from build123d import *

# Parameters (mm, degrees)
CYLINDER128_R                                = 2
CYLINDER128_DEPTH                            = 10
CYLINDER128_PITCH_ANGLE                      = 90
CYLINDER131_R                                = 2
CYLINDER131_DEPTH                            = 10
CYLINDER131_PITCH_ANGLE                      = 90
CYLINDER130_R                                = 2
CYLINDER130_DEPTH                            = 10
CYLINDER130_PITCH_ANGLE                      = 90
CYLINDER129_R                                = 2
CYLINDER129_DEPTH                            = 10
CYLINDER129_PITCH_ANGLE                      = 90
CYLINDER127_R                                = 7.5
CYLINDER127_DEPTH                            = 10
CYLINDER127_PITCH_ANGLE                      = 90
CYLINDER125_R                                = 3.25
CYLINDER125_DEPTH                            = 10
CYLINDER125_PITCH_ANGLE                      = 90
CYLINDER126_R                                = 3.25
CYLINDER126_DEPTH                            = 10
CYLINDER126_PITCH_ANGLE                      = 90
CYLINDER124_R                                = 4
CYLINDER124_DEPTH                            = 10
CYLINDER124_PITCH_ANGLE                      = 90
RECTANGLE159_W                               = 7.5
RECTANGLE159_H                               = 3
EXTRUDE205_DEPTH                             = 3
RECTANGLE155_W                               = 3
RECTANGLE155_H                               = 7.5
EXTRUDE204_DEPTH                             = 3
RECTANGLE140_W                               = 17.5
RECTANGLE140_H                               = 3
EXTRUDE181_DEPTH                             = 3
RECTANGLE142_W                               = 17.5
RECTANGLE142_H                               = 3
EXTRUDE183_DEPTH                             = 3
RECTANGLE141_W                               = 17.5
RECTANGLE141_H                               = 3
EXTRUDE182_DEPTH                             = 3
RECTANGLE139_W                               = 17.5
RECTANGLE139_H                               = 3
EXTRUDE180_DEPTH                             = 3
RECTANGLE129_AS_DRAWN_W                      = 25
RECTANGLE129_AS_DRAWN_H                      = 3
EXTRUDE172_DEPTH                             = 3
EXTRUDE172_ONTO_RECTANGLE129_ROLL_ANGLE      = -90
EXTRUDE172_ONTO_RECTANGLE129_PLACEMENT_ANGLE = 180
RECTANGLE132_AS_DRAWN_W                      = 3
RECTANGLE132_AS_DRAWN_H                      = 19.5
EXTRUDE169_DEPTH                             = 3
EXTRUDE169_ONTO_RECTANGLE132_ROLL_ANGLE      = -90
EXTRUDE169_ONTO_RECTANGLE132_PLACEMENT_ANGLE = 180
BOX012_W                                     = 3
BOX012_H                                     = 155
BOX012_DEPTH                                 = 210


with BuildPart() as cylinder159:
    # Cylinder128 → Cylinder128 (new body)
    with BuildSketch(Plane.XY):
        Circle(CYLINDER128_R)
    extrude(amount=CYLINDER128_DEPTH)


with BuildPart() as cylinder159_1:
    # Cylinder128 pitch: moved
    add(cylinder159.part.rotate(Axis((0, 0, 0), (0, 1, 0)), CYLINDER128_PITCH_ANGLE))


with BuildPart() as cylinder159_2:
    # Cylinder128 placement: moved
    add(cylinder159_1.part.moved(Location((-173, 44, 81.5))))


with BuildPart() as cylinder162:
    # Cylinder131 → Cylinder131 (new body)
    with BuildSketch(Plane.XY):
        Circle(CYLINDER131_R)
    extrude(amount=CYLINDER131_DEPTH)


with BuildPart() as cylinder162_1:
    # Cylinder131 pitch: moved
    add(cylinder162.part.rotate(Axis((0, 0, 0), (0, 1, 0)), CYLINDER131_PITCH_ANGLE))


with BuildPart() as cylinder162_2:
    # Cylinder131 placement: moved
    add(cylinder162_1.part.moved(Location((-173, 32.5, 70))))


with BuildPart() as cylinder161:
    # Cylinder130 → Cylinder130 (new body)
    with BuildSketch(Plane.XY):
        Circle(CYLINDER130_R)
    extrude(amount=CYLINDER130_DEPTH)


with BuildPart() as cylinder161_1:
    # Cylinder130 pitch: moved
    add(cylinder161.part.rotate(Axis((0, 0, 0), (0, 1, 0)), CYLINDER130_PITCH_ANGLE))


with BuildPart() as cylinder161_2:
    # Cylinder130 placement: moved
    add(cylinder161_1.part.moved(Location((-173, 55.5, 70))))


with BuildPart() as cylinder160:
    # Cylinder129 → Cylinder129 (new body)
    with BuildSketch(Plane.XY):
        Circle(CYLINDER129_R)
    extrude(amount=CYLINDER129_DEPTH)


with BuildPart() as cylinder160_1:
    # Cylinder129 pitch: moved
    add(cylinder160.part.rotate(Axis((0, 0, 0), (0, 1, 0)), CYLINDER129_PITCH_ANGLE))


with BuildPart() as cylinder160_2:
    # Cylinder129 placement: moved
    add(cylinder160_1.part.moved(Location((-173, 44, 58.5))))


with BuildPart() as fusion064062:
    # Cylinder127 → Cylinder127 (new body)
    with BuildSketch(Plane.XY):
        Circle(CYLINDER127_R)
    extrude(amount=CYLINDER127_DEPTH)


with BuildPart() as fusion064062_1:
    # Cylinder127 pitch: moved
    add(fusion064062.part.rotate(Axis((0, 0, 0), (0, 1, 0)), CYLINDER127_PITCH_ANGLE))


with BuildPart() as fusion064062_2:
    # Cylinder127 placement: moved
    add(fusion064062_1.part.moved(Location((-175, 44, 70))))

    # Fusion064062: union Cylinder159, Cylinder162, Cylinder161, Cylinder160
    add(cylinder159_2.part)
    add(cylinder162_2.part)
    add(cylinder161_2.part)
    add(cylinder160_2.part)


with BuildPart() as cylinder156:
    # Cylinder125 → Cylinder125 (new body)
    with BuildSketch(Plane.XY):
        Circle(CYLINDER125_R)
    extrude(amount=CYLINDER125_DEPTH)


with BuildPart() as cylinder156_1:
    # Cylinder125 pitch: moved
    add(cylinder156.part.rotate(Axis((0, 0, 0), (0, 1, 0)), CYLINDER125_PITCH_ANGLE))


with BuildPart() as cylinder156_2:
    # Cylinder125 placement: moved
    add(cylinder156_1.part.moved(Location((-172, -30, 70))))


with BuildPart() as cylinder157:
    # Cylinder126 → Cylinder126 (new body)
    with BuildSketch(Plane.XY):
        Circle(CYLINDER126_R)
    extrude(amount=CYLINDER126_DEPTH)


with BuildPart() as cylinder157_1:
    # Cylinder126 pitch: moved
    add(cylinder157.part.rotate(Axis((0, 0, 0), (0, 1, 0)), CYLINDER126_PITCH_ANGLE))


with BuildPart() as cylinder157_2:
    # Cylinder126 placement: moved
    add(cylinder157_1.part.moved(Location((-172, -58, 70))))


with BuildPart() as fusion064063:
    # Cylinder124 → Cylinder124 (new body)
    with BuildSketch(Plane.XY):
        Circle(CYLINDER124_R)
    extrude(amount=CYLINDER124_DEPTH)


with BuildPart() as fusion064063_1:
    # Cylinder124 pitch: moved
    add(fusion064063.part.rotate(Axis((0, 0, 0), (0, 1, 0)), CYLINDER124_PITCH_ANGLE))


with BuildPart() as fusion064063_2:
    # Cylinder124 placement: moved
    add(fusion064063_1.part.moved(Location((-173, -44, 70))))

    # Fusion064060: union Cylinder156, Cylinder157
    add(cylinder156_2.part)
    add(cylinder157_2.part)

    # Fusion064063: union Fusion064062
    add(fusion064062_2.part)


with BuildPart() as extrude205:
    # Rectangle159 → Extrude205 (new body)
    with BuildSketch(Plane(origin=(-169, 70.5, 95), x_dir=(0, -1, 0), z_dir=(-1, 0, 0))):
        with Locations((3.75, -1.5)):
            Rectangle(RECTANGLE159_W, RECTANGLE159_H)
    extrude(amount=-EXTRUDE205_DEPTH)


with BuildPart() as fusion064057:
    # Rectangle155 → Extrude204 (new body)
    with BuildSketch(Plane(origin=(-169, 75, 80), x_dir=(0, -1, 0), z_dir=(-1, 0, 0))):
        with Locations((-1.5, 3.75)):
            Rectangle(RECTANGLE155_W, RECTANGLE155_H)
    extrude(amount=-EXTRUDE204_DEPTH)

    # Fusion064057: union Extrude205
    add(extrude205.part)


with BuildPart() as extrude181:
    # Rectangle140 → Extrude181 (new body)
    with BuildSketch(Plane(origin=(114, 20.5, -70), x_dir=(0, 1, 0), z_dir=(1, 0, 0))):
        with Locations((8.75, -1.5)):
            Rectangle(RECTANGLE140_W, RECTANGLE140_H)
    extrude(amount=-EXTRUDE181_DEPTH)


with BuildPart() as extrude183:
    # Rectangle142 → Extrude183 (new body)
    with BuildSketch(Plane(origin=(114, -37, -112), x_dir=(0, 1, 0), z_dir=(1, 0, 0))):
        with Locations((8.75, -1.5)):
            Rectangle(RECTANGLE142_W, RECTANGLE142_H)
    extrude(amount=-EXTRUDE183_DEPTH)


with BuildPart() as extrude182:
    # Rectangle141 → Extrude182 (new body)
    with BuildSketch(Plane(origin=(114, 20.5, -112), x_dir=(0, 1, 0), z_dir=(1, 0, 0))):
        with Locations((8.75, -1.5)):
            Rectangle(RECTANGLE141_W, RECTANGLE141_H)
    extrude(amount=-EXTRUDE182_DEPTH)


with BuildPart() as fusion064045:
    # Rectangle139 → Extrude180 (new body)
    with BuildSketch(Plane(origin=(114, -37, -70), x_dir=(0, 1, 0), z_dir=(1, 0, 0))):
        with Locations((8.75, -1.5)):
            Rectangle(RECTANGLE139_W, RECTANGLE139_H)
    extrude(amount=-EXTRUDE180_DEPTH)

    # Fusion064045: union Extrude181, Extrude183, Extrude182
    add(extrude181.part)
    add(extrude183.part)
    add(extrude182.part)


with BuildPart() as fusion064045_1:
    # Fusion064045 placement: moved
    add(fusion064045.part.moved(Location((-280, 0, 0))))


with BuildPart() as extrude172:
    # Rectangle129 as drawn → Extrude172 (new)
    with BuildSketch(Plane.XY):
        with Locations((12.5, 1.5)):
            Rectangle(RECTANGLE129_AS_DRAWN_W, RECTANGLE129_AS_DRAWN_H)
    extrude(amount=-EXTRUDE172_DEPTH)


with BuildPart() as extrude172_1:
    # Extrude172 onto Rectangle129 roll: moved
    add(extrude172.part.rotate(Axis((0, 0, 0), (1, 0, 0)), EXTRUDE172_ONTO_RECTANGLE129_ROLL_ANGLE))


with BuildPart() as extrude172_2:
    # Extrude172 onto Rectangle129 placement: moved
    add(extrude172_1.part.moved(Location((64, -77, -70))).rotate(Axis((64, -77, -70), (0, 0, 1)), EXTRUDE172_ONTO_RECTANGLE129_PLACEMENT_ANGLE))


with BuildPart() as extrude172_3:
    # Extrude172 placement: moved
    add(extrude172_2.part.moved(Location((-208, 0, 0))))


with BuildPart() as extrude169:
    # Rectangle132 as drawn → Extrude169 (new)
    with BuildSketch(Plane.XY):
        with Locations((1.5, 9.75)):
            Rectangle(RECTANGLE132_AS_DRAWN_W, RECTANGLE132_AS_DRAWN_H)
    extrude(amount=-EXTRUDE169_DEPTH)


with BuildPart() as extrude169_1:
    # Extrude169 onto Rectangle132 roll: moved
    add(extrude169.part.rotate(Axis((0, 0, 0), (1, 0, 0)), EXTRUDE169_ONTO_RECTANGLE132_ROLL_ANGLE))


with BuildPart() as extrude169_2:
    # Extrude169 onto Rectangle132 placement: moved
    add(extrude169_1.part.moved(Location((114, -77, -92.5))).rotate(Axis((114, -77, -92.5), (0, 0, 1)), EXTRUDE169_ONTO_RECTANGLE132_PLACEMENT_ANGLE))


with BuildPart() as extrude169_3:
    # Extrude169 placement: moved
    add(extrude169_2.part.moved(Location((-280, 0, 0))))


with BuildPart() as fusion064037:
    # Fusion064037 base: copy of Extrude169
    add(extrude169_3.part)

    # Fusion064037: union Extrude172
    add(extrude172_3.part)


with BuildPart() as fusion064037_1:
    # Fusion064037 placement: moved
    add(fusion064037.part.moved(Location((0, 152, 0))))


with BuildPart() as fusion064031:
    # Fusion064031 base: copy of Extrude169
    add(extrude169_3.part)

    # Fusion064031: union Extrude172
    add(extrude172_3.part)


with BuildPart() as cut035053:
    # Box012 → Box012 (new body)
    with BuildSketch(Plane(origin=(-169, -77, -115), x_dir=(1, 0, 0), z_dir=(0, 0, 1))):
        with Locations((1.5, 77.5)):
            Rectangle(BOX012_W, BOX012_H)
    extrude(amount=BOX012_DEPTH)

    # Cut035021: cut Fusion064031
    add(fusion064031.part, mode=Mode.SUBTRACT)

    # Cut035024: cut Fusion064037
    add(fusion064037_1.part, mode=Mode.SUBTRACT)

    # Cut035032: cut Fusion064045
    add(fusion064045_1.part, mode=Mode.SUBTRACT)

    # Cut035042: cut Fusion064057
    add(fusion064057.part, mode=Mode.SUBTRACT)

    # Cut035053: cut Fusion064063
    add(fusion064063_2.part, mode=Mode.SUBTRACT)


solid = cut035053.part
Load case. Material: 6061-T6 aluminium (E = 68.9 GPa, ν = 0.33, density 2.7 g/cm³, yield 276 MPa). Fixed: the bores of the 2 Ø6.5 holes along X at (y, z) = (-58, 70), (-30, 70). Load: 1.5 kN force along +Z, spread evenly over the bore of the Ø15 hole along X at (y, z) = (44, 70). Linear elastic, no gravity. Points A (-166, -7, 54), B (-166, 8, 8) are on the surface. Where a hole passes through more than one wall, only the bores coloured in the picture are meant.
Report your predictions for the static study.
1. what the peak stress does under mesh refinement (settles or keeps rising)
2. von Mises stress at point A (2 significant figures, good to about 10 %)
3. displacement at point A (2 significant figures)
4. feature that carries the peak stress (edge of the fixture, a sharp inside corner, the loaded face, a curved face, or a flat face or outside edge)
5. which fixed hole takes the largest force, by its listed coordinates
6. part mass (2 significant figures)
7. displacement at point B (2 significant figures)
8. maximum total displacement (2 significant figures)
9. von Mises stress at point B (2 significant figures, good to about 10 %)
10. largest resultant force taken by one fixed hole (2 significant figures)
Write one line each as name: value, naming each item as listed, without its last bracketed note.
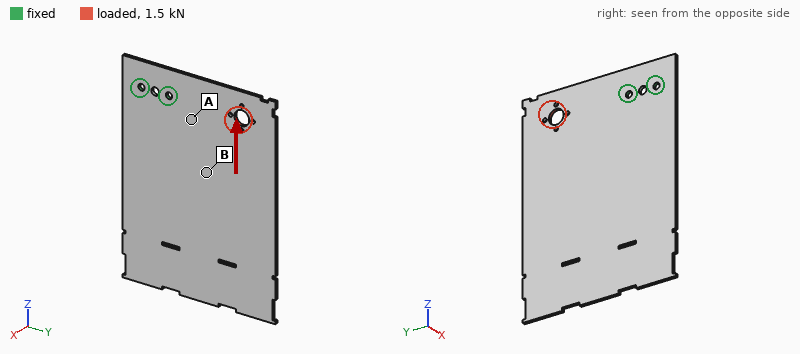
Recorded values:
what the peak stress does under mesh refinement: keeps rising
von Mises stress at point A: 17 MPa
displacement at point A: 0.047 mm
feature that carries the peak stress: edge of the fixture
which fixed hole takes the largest force, by its listed coordinates: (-30, 70)
part mass: 260 g
displacement at point B: 0.11 mm
maximum total displacement: 0.29 mm
von Mises stress at point B: 6.6 MPa
largest resultant force taken by one fixed hole: 4.8 kN
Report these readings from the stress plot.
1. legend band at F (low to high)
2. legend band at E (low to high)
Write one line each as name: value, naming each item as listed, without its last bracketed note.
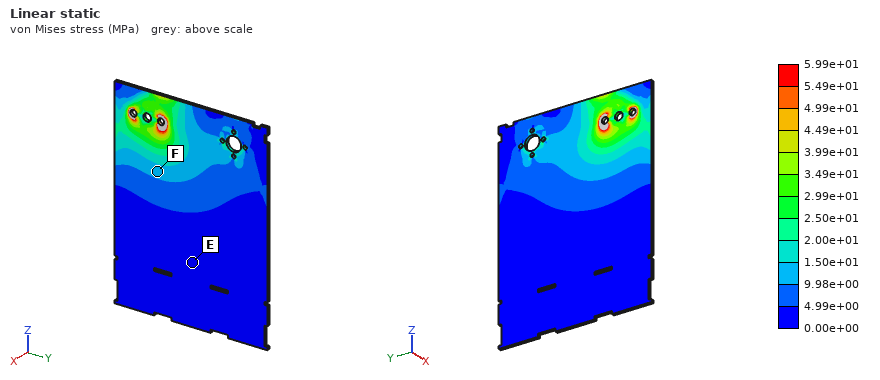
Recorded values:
legend band at F: 9.98e+00 to 1.50e+01 MPa
legend band at E: 0.00e+00 to 4.99e+00 MPa
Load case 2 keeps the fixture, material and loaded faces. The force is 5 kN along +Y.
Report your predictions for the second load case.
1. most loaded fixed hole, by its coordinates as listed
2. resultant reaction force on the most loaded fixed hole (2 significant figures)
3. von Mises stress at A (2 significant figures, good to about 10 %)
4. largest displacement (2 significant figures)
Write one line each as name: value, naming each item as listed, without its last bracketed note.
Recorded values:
most loaded fixed hole, by its coordinates as listed: (-30, 70)
resultant reaction force on the most loaded fixed hole: 3.6 kN
von Mises stress at A: 22 MPa
largest displacement: 53 µm
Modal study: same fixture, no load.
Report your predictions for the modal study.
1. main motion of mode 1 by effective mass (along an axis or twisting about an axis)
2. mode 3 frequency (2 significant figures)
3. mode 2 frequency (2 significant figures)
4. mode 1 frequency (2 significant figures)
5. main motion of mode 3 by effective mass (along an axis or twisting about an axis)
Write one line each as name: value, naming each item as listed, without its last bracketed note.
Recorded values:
main motion of mode 1 by effective mass: along X
mode 3 frequency: 300 Hz
mode 2 frequency: 140 Hz
mode 1 frequency: 60 Hz
main motion of mode 3 by effective mass: along X
